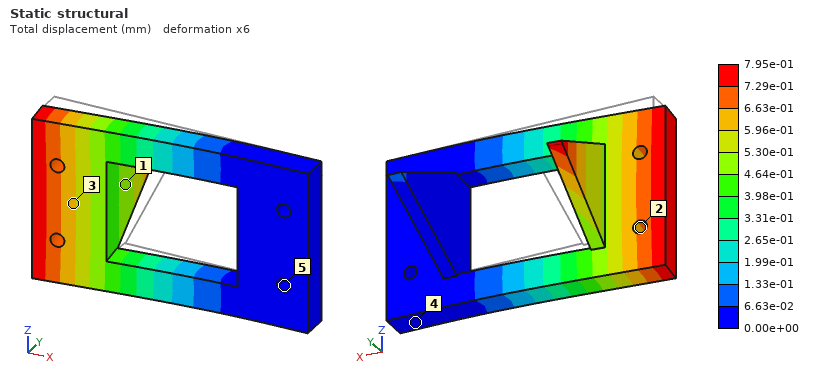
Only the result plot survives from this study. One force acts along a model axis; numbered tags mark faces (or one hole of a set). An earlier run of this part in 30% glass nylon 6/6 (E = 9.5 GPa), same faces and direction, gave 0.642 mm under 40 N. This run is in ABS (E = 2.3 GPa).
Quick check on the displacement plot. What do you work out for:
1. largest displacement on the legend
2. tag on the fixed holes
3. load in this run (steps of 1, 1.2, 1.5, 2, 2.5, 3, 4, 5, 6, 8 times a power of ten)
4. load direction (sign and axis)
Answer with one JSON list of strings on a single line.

["7.95e-01 mm", "5", "12 N", "-Y"]
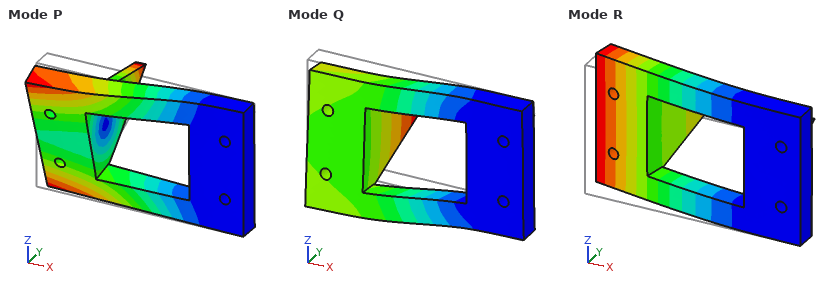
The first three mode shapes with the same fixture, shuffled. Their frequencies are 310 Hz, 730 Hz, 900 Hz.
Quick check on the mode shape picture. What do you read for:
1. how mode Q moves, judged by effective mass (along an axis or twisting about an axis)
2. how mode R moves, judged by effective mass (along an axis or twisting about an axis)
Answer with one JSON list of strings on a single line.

["along Z", "along Y"]
